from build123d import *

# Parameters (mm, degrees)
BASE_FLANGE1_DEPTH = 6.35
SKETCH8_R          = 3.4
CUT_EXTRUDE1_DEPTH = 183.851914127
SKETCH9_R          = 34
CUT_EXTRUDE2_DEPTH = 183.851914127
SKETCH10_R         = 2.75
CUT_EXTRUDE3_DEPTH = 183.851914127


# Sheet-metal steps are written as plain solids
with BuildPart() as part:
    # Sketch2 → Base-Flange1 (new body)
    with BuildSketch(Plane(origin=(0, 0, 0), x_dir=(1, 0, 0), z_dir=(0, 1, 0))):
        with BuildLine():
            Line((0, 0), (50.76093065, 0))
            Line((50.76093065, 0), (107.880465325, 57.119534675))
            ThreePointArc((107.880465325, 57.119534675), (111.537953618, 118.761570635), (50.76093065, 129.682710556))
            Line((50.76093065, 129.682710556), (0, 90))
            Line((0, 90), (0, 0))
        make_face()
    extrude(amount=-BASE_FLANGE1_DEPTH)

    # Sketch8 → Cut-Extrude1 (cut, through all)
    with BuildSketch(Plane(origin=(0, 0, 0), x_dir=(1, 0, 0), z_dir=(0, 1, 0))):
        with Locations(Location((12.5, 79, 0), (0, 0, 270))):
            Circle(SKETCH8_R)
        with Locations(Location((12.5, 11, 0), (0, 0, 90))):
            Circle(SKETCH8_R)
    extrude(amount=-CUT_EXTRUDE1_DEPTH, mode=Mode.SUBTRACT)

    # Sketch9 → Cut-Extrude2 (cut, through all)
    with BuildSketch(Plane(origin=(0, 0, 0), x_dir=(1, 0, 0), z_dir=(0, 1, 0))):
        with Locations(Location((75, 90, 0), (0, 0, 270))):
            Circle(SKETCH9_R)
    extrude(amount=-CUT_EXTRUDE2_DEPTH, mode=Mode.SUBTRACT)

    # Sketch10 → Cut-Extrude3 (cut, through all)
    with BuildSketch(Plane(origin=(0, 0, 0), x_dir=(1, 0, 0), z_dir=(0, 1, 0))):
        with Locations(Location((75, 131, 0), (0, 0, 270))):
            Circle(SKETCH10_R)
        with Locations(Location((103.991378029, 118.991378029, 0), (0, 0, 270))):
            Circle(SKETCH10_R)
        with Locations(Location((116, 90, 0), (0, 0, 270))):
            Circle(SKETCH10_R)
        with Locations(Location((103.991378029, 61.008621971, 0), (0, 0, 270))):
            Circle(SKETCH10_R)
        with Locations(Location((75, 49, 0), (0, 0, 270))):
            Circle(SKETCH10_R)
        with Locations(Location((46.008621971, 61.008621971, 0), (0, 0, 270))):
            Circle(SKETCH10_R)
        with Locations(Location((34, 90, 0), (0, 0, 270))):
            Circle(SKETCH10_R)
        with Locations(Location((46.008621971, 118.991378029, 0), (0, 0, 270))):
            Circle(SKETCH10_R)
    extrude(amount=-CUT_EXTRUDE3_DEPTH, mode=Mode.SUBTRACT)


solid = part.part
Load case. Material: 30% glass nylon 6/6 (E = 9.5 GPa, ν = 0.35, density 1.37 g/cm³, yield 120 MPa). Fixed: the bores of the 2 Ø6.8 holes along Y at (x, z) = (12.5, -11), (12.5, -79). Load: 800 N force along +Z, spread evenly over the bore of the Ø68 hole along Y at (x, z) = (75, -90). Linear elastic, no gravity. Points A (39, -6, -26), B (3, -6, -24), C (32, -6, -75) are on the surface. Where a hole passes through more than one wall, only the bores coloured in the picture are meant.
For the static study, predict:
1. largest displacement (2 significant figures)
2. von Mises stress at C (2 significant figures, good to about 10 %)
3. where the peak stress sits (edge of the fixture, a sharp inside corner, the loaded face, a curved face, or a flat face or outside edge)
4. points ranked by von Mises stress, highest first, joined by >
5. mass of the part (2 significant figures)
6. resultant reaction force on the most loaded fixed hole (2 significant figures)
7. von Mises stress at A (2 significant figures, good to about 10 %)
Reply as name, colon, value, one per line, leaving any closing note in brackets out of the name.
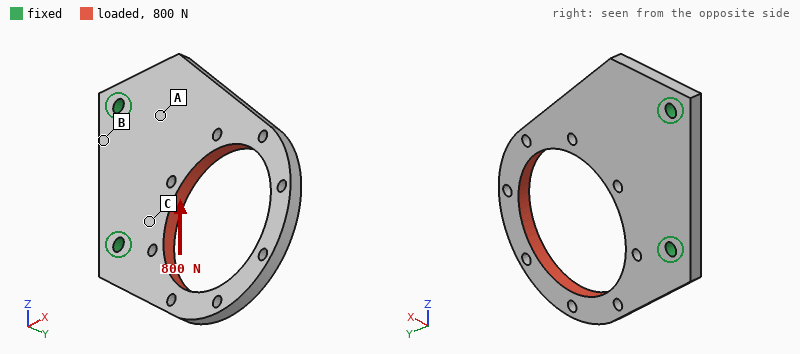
largest displacement: 0.32 mm
von Mises stress at C: 5.8 MPa
where the peak stress sits: a curved face
points ranked by von Mises stress, highest first, joined by >: C > A > B
mass of the part: 72 g
resultant reaction force on the most loaded fixed hole: 820 N
von Mises stress at A: 3.0 MPa
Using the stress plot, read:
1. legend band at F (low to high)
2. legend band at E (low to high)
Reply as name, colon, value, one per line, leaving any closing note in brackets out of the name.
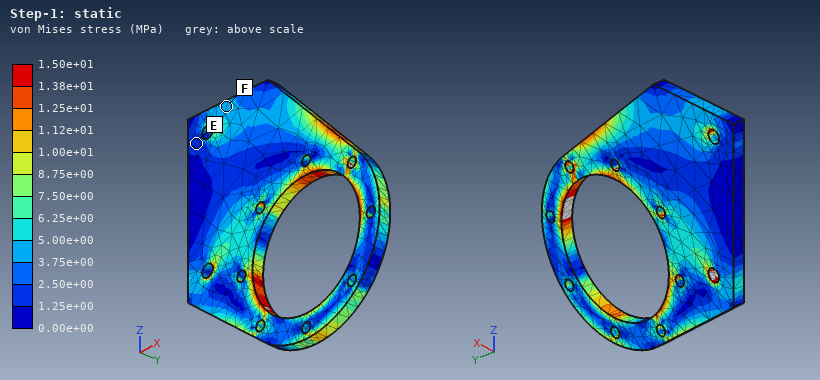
legend band at F: 3.75e+00 to 5.00e+00 MPa
legend band at E: 1.25e+00 to 2.50e+00 MPa
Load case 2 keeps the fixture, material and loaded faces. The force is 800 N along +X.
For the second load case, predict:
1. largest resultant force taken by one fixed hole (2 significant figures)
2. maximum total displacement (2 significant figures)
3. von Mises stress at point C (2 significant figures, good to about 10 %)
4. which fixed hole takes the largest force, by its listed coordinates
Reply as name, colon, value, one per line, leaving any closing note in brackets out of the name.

largest resultant force taken by one fixed hole: 900 N
maximum total displacement: 0.27 mm
von Mises stress at point C: 4.6 MPa
which fixed hole takes the largest force, by its listed coordinates: (12.5, -79)
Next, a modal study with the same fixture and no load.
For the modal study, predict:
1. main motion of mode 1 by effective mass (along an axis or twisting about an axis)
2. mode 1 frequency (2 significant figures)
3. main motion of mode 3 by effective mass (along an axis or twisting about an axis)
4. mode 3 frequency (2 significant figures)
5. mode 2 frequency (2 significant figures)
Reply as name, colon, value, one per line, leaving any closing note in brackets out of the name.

main motion of mode 1 by effective mass: along Y
mode 1 frequency: 260 Hz
main motion of mode 3 by effective mass: along Y
mode 3 frequency: 1000 Hz
mode 2 frequency: 540 Hz
